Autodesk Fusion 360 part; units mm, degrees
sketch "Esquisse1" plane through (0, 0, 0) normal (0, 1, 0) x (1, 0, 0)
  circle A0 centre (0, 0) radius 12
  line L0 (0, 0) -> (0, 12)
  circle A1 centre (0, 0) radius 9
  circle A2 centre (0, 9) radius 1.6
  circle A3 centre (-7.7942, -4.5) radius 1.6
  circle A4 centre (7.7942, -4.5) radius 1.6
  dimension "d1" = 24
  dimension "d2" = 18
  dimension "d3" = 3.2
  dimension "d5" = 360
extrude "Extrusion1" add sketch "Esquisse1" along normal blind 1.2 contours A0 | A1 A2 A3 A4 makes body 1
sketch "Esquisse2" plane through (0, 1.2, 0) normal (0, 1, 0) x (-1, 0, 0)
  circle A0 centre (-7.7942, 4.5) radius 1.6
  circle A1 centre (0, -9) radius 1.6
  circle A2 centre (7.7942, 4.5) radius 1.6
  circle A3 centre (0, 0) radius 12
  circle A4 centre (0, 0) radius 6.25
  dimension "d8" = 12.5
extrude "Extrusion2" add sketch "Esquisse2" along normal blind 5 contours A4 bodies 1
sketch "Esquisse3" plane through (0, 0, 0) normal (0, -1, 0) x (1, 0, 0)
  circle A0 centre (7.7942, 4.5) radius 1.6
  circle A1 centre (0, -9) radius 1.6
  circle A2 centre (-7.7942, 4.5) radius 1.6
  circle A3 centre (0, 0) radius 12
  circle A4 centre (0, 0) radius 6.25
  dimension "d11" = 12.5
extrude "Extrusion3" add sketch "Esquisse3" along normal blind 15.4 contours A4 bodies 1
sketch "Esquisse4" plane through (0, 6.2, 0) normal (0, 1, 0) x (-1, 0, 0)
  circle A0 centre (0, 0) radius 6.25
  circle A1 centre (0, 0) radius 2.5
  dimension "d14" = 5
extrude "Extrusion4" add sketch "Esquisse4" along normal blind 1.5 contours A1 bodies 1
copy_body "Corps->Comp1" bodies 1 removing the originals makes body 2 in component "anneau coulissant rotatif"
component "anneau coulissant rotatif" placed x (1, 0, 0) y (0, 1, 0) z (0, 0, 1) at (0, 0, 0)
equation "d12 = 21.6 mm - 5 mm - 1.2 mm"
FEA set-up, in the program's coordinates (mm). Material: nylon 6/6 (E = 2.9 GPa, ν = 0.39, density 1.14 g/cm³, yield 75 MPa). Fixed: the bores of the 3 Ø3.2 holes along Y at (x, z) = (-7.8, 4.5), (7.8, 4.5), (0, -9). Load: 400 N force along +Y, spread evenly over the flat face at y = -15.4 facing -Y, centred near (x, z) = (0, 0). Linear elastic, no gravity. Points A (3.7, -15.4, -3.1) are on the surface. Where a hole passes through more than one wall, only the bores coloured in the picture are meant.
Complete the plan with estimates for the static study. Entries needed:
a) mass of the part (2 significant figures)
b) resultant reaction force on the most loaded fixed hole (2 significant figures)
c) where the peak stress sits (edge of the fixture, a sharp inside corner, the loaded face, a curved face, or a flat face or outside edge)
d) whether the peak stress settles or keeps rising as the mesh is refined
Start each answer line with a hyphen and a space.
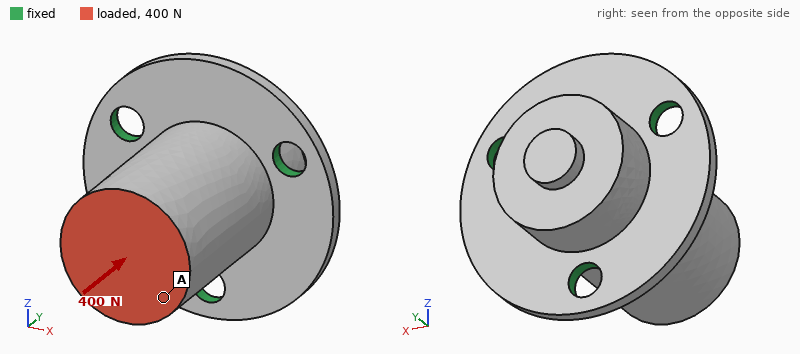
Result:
- 3.5 g
- 130 N
- edge of the fixture
- keeps rising
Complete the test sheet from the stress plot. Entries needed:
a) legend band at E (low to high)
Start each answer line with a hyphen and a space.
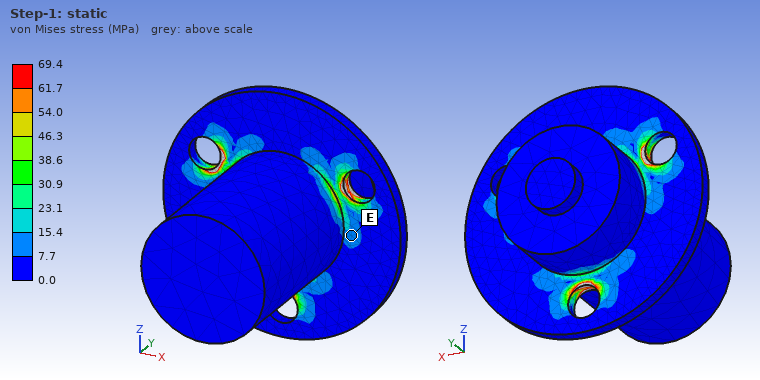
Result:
- 7.7 to 15.4 MPa
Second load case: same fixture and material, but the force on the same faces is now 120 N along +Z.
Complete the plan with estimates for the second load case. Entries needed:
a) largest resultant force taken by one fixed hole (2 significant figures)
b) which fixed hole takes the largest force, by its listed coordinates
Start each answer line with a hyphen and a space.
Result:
- 180 N
- (0, -9)
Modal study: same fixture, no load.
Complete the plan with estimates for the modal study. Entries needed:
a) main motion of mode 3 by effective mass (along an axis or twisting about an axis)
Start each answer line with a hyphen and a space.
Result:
- along Y
